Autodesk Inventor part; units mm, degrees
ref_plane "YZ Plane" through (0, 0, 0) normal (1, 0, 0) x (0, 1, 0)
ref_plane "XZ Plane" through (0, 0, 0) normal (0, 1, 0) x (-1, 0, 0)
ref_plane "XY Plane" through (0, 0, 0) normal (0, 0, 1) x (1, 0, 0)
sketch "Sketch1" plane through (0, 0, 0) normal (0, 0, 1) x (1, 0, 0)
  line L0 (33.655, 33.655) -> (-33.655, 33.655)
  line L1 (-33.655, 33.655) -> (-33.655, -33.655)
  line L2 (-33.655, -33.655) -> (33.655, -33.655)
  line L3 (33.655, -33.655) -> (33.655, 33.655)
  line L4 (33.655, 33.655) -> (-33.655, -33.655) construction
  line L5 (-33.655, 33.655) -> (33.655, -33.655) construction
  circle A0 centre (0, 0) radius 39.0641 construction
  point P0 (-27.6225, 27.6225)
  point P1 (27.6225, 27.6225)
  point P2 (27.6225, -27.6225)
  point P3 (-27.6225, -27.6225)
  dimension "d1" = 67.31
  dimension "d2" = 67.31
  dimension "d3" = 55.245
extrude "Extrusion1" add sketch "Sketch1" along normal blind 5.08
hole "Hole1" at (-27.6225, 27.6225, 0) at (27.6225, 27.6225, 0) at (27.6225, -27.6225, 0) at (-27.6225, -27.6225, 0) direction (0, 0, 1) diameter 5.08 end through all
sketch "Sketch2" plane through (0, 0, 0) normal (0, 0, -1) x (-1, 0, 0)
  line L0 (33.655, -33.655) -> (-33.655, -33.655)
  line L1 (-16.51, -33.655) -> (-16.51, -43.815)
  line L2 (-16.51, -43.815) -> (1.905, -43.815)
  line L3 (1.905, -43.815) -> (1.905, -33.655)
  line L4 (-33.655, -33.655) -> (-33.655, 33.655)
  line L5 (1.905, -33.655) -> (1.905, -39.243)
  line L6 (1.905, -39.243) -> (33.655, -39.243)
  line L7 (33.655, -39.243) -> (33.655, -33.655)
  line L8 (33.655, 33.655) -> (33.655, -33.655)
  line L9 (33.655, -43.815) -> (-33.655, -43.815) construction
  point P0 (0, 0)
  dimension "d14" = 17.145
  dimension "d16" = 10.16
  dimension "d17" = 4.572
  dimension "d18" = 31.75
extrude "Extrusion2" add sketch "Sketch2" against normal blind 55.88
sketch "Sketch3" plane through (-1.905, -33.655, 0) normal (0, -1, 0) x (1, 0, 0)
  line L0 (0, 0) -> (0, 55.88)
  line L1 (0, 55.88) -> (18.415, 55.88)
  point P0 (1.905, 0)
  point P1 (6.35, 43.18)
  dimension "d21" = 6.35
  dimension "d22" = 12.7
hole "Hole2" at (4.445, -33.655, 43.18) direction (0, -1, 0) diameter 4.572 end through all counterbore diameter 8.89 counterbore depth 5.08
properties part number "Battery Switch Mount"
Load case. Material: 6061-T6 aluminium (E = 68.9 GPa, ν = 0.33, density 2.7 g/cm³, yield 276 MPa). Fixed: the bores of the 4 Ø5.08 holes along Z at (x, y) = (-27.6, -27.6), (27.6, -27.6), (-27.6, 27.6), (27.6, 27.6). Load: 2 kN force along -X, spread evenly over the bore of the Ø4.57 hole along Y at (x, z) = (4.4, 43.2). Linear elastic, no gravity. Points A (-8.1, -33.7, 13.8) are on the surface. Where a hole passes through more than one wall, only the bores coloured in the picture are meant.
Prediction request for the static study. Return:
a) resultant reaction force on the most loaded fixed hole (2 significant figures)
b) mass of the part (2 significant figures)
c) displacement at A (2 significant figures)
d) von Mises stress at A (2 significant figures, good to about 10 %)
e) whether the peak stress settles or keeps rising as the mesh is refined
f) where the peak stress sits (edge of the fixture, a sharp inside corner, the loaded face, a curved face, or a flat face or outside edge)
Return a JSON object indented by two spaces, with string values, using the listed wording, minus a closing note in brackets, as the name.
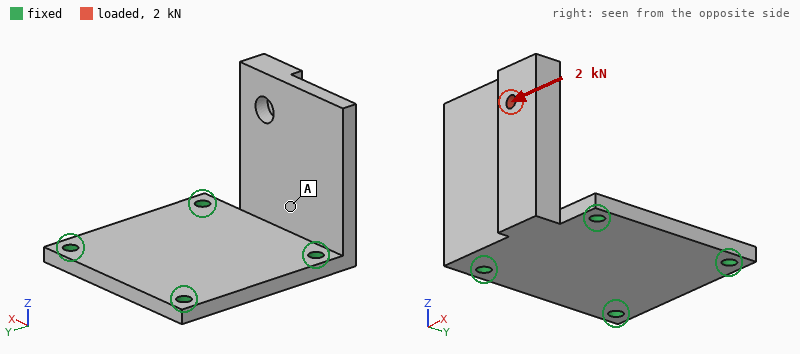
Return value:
{
  "resultant reaction force on the most loaded fixed hole": "2.0 kN",
  "mass of the part": "110 g",
  "displacement at A": "0.052 mm",
  "von Mises stress at A": "20 MPa",
  "whether the peak stress settles or keeps rising as the mesh is refined": "keeps rising",
  "where the peak stress sits": "a sharp inside corner"
}
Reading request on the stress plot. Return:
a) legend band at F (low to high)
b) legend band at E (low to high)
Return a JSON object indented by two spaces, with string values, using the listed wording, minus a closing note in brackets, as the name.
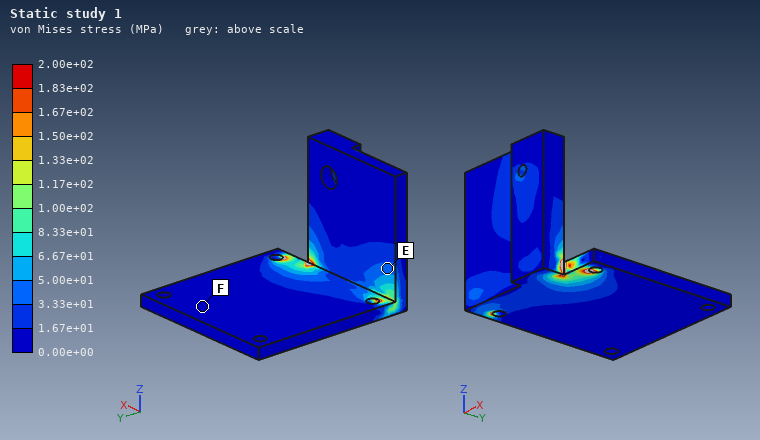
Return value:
{
  "legend band at F": "0.00e+00 to 1.67e+01 MPa",
  "legend band at E": "3.33e+01 to 5.00e+01 MPa"
}
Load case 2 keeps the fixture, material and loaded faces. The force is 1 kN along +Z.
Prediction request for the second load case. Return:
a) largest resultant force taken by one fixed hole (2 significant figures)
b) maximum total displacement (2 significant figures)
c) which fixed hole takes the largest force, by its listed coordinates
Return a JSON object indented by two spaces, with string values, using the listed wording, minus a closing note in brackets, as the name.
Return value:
{
  "largest resultant force taken by one fixed hole": "690 N",
  "maximum total displacement": "0.27 mm",
  "which fixed hole takes the largest force, by its listed coordinates": "(27.6, -27.6)"
}
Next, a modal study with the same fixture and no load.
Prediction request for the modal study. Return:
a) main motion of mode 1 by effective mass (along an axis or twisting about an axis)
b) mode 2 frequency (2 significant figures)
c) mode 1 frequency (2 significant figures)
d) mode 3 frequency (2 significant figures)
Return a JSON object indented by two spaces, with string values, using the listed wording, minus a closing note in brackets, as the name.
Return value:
{
  "main motion of mode 1 by effective mass": "along Y",
  "mode 2 frequency": "3100 Hz",
  "mode 1 frequency": "1100 Hz",
  "mode 3 frequency": "4300 Hz"
}
